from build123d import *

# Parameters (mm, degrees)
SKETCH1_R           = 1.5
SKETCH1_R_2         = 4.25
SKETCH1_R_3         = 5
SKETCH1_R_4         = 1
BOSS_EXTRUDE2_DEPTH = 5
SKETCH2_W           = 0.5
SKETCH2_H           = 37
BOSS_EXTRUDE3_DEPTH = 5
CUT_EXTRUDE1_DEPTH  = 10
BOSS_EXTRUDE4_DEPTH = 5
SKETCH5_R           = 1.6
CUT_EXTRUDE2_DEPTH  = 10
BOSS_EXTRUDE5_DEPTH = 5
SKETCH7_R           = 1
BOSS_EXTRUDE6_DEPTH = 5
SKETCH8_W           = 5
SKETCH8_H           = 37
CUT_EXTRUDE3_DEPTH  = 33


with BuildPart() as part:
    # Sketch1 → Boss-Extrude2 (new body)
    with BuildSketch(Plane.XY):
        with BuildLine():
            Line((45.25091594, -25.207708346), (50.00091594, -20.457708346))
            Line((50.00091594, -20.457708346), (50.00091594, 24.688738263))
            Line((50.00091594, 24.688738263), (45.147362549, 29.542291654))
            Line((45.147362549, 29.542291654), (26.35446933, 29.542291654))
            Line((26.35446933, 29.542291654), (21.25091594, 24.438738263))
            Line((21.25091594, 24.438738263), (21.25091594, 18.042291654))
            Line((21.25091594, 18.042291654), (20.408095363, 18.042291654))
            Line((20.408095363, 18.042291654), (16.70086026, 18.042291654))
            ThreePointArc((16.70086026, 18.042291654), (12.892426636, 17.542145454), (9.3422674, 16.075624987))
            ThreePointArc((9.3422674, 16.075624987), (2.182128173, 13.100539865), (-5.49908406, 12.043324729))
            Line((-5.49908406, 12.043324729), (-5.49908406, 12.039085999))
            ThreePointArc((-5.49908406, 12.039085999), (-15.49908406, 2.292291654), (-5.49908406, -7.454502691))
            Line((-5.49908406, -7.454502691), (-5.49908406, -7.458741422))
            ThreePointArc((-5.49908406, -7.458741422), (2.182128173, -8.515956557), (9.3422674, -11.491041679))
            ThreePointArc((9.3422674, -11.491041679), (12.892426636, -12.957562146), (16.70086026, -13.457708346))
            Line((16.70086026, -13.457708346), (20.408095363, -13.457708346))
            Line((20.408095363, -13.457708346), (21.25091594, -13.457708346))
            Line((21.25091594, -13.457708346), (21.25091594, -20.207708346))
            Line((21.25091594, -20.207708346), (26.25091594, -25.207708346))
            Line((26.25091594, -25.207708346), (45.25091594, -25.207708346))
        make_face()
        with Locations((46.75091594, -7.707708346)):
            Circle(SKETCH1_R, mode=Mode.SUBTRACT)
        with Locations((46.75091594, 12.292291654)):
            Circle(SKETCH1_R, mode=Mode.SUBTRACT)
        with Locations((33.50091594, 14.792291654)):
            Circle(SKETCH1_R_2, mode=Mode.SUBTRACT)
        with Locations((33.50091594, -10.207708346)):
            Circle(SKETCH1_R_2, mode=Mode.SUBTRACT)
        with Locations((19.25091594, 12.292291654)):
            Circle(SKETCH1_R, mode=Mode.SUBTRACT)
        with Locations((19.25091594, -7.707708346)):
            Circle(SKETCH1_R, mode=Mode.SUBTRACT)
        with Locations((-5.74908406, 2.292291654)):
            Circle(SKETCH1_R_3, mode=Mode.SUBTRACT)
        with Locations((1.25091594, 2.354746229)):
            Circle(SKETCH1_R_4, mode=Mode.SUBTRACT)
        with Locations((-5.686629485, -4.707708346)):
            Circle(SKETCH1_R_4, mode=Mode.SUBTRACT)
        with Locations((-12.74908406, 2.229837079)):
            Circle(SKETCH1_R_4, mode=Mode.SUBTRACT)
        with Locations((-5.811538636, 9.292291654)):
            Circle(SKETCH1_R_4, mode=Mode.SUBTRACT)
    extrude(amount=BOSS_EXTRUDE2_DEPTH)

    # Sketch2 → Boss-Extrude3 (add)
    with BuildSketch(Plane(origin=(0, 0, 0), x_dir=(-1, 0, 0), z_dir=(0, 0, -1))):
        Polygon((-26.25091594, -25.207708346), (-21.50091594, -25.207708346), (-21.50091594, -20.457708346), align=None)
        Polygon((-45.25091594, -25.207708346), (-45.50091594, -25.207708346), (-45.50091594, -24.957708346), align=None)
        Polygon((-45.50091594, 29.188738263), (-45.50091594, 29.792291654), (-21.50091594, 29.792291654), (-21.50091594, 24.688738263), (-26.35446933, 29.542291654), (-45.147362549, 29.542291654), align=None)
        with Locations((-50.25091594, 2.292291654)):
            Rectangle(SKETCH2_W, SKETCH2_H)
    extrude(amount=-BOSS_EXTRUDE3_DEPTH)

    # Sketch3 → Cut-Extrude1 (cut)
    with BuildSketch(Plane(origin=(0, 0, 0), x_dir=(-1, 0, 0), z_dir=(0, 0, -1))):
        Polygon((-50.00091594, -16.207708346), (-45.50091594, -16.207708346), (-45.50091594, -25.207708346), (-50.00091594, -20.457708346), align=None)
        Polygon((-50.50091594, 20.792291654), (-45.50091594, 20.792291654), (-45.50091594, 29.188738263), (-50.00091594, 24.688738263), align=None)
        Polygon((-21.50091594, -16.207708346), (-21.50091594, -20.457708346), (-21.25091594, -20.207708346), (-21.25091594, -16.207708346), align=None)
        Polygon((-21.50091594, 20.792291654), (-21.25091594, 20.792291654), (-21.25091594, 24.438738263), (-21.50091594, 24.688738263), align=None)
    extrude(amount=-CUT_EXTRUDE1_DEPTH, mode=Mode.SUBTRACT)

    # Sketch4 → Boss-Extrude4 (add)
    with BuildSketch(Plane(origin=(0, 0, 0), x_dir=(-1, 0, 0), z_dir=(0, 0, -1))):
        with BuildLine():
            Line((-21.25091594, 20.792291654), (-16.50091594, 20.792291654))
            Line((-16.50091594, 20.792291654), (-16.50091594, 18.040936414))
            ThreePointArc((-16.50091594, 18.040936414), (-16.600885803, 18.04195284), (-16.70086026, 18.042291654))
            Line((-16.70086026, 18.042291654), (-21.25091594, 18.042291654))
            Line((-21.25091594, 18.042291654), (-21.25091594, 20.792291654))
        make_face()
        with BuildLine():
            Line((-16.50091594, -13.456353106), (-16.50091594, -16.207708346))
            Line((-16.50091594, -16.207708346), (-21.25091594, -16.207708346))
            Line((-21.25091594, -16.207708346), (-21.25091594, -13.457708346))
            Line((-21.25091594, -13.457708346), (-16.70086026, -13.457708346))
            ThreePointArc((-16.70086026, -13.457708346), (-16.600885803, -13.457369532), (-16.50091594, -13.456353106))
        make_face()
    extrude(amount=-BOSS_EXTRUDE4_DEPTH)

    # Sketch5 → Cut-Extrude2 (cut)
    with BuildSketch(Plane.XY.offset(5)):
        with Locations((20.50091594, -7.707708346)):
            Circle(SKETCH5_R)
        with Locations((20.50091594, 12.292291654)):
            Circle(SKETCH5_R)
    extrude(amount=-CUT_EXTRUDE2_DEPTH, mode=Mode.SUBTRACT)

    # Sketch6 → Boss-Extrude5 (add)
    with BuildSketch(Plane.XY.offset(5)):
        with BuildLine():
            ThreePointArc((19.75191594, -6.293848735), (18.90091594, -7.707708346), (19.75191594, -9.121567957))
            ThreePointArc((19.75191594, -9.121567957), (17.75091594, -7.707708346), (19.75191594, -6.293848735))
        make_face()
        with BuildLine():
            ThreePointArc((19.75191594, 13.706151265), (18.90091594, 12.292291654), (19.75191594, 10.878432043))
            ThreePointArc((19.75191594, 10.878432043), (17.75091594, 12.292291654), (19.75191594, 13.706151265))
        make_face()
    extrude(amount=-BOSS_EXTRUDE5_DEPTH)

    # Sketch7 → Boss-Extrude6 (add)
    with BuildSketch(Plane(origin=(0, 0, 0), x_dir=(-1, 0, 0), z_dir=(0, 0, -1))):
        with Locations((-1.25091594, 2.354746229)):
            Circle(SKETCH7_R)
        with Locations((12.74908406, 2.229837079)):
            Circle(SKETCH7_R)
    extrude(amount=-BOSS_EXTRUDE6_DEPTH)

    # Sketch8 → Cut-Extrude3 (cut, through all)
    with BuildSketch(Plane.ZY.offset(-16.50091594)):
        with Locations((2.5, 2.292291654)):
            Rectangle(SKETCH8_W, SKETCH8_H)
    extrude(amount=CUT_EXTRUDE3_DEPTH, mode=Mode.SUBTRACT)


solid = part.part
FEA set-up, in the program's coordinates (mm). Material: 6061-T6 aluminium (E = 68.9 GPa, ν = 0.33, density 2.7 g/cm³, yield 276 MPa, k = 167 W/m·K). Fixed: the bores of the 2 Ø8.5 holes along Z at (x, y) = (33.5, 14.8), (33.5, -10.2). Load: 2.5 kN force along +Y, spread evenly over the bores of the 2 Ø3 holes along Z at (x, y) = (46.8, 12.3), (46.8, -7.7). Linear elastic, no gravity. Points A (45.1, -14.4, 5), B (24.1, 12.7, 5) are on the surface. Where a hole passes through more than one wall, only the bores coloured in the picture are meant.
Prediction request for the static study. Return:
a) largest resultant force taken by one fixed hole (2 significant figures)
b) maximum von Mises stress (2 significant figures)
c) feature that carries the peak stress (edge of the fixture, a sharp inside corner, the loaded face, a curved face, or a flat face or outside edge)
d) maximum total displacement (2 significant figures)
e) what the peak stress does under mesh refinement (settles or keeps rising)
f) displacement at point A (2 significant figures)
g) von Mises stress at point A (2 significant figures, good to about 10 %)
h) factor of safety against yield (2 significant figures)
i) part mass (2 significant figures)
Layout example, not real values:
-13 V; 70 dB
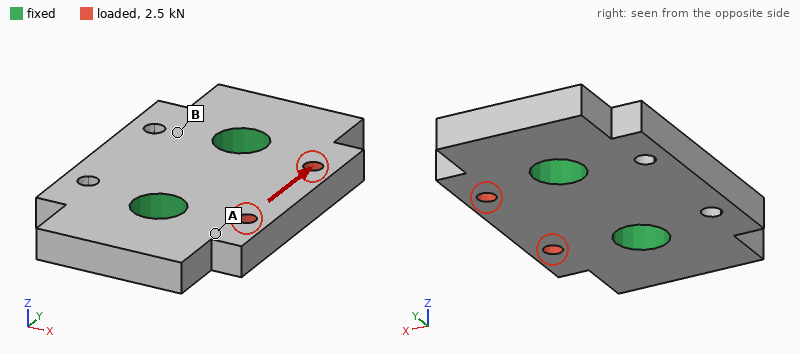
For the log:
1.5 kN; 52 MPa; the loaded face; 8.0 µm; settles; 4.9 µm; 16 MPa; 5.3; 21 g
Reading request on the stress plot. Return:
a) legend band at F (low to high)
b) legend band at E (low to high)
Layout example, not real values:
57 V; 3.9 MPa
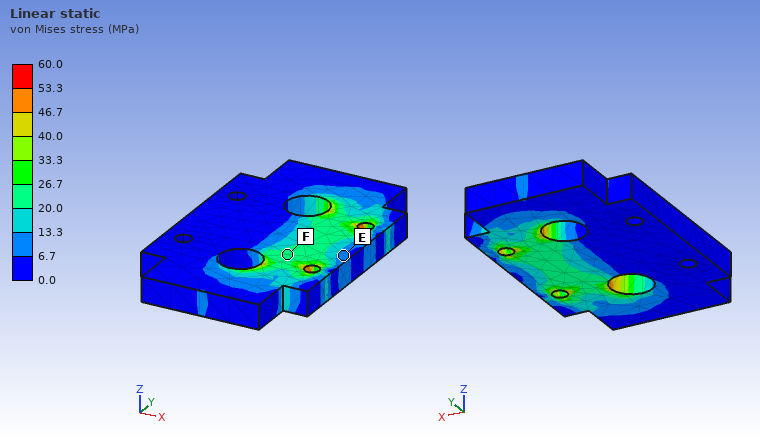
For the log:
20.0 to 26.7 MPa; 6.7 to 13.3 MPa
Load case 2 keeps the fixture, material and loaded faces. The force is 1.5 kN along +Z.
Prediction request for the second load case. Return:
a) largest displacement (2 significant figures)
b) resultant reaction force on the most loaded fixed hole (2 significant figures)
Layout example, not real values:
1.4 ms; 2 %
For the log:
38 µm; 750 N
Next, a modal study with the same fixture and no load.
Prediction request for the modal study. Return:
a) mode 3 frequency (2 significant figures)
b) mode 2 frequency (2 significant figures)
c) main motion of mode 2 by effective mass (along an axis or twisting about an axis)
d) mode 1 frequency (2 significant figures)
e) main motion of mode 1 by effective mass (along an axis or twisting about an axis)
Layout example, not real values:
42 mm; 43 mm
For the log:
22 kHz; 20 kHz; along Z; 18 kHz; twisting about Y
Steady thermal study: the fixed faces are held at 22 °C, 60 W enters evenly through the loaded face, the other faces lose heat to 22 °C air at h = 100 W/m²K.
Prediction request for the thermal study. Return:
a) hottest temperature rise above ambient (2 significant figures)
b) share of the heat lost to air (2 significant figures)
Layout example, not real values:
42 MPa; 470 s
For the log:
28 K; 3.8 %
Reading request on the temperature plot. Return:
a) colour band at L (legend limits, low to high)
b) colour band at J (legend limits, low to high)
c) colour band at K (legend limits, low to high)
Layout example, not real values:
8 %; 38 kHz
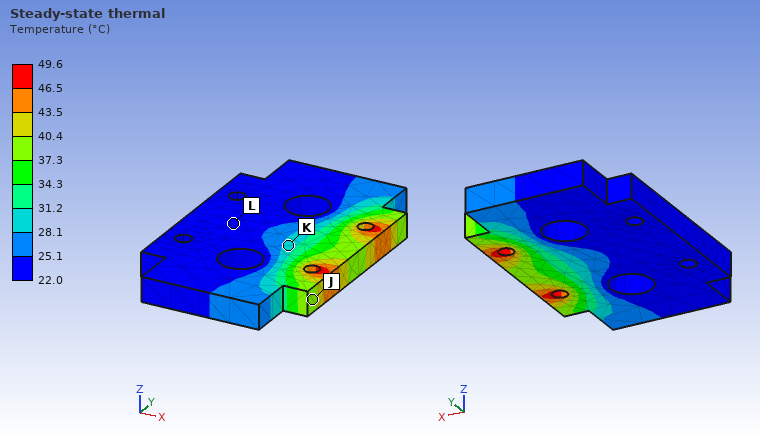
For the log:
22.0 to 25.1 °C; 37.3 to 40.4 °C; 28.1 to 31.2 °C
